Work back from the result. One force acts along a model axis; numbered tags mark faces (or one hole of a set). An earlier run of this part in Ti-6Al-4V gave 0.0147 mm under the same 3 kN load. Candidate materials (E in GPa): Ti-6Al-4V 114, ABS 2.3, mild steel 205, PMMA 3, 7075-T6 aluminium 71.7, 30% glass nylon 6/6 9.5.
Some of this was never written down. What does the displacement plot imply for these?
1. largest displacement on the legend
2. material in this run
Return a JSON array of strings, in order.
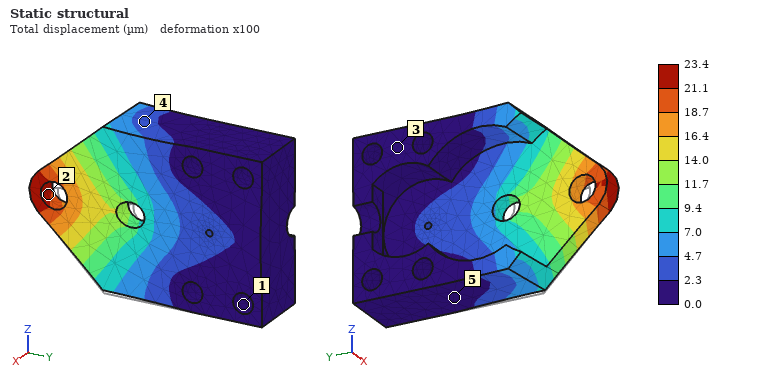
["23.4 µm", "7075-T6 aluminium"]
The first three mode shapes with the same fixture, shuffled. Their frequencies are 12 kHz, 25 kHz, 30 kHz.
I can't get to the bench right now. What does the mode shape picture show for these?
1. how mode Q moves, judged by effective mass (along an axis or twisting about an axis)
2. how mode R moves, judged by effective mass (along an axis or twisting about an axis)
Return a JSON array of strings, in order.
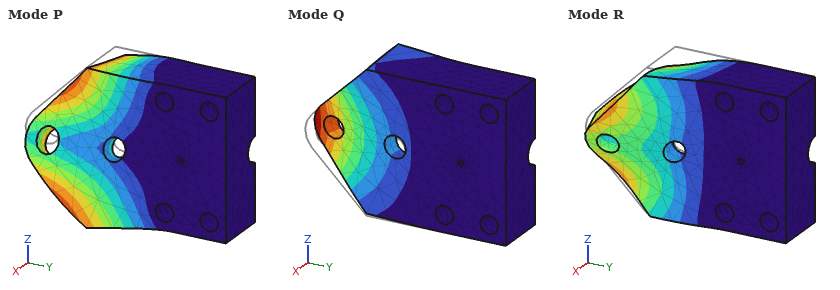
["along X", "along Z"]
